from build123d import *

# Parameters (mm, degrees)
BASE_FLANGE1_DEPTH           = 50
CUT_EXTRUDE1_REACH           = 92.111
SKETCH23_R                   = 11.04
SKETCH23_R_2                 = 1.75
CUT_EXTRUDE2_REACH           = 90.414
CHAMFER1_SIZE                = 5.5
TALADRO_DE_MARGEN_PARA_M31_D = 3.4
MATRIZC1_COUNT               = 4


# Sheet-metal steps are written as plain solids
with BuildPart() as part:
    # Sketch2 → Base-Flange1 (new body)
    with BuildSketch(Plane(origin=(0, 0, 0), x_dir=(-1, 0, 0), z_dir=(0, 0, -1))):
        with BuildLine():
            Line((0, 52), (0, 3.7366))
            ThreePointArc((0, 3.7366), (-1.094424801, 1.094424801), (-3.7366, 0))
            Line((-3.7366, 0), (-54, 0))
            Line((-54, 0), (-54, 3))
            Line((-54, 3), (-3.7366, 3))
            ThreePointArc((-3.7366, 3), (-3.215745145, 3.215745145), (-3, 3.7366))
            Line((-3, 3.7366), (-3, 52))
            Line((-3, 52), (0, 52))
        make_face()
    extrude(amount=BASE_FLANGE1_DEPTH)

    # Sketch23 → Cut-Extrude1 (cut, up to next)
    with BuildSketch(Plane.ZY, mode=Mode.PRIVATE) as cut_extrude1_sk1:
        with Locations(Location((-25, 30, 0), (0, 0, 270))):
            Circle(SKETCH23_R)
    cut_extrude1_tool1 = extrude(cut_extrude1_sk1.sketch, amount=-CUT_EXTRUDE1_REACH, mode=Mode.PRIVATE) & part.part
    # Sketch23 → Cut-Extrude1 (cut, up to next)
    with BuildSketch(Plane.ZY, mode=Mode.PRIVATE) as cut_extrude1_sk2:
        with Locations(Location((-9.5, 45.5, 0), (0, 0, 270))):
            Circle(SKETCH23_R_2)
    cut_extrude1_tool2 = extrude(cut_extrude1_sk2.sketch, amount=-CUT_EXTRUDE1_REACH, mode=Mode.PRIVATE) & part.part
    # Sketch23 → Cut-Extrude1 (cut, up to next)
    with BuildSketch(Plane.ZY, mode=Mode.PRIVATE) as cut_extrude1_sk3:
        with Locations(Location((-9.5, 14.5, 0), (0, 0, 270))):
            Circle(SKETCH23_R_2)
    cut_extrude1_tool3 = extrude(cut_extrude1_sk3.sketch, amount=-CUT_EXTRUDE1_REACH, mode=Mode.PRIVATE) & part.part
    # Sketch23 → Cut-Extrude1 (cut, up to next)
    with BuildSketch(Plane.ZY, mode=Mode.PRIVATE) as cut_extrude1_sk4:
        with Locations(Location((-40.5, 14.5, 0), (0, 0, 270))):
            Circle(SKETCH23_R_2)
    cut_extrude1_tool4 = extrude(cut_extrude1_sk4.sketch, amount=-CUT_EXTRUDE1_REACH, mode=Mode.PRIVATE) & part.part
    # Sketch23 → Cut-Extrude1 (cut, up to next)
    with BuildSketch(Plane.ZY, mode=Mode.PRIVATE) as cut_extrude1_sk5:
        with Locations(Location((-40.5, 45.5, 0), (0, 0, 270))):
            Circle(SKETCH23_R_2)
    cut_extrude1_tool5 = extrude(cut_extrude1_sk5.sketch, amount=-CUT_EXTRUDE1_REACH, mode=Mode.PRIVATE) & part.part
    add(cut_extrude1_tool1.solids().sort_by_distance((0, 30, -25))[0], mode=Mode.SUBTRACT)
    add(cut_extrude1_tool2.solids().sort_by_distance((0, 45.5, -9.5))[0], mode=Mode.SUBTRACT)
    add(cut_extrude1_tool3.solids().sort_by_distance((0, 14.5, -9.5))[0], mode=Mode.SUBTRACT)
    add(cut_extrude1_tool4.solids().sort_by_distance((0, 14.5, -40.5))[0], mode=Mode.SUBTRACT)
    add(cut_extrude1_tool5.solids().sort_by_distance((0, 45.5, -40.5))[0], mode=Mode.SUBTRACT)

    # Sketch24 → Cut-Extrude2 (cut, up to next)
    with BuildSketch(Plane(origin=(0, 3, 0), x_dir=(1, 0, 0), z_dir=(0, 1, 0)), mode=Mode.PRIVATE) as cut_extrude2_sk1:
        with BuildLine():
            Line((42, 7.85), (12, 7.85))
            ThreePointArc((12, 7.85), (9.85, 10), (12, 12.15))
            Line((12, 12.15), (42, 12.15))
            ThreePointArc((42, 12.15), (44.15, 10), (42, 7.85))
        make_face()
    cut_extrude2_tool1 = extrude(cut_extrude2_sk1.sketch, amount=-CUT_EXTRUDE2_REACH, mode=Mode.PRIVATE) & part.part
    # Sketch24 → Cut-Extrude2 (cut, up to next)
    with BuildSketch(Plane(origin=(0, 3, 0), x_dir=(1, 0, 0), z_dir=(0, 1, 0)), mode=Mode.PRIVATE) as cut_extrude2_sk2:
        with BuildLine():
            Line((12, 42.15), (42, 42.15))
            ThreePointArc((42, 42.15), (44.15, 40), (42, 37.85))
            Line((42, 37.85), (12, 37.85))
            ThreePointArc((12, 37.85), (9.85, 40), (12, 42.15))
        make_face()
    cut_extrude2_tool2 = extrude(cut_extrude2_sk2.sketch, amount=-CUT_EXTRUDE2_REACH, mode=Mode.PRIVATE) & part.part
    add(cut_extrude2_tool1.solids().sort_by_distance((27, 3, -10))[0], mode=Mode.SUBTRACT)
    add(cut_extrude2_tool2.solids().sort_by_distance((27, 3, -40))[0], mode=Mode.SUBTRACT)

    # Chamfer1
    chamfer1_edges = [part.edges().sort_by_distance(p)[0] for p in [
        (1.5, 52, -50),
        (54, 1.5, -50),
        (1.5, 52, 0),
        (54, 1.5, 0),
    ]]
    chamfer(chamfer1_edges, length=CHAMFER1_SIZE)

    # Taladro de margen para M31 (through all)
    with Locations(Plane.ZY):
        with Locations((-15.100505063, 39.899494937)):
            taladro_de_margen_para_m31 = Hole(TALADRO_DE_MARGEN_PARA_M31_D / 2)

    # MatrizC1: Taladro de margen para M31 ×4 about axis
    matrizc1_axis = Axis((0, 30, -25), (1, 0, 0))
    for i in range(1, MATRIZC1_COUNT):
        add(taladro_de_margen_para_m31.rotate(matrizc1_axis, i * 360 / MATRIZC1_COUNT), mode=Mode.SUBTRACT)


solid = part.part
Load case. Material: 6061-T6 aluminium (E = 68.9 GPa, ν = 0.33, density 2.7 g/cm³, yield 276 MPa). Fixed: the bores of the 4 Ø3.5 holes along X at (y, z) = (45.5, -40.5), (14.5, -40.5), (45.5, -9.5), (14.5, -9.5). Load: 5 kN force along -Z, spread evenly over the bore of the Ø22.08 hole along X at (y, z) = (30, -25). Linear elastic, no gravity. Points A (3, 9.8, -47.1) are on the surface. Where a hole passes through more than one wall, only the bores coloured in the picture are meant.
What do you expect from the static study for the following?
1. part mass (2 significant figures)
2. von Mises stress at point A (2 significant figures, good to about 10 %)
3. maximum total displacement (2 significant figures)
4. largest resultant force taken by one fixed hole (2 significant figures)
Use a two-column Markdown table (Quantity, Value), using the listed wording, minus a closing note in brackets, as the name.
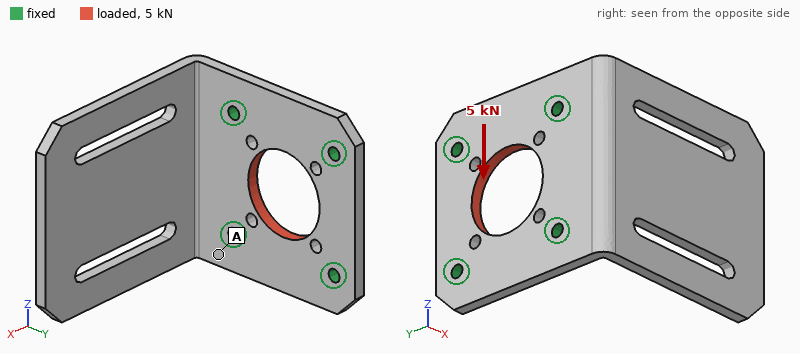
| Quantity | Value |
|---|---|
| part mass | 35 g |
| von Mises stress at point A | 9.1 MPa |
| maximum total displacement | 12 µm |
| largest resultant force taken by one fixed hole | 1.3 kN |
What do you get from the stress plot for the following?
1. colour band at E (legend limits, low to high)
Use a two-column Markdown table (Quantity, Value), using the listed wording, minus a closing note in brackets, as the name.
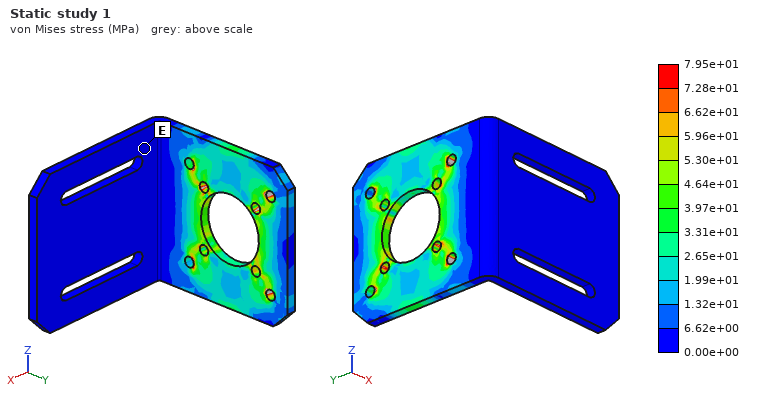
| Quantity | Value |
|---|---|
| colour band at E | 0.00e+00 to 6.62e+00 MPa |
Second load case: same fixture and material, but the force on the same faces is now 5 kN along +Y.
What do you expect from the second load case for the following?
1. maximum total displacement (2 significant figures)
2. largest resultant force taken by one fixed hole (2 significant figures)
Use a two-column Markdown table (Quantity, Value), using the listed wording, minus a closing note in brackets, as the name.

| Quantity | Value |
|---|---|
| maximum total displacement | 15 µm |
| largest resultant force taken by one fixed hole | 1.3 kN |
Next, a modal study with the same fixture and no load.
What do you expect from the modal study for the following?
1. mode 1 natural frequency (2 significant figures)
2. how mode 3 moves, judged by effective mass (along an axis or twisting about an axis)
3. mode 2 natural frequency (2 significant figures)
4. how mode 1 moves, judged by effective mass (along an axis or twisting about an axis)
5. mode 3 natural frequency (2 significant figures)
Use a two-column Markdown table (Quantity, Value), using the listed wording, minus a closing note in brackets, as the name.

| Quantity | Value |
|---|---|
| mode 1 natural frequency | 660 Hz |
| how mode 3 moves, judged by effective mass | along Z |
| mode 2 natural frequency | 1800 Hz |
| how mode 1 moves, judged by effective mass | along Y |
| mode 3 natural frequency | 2500 Hz |
